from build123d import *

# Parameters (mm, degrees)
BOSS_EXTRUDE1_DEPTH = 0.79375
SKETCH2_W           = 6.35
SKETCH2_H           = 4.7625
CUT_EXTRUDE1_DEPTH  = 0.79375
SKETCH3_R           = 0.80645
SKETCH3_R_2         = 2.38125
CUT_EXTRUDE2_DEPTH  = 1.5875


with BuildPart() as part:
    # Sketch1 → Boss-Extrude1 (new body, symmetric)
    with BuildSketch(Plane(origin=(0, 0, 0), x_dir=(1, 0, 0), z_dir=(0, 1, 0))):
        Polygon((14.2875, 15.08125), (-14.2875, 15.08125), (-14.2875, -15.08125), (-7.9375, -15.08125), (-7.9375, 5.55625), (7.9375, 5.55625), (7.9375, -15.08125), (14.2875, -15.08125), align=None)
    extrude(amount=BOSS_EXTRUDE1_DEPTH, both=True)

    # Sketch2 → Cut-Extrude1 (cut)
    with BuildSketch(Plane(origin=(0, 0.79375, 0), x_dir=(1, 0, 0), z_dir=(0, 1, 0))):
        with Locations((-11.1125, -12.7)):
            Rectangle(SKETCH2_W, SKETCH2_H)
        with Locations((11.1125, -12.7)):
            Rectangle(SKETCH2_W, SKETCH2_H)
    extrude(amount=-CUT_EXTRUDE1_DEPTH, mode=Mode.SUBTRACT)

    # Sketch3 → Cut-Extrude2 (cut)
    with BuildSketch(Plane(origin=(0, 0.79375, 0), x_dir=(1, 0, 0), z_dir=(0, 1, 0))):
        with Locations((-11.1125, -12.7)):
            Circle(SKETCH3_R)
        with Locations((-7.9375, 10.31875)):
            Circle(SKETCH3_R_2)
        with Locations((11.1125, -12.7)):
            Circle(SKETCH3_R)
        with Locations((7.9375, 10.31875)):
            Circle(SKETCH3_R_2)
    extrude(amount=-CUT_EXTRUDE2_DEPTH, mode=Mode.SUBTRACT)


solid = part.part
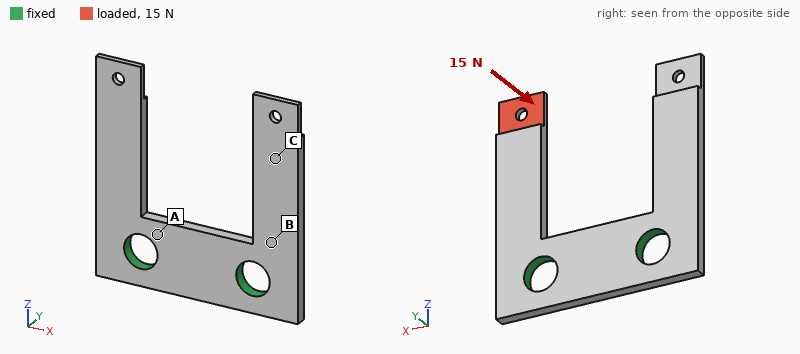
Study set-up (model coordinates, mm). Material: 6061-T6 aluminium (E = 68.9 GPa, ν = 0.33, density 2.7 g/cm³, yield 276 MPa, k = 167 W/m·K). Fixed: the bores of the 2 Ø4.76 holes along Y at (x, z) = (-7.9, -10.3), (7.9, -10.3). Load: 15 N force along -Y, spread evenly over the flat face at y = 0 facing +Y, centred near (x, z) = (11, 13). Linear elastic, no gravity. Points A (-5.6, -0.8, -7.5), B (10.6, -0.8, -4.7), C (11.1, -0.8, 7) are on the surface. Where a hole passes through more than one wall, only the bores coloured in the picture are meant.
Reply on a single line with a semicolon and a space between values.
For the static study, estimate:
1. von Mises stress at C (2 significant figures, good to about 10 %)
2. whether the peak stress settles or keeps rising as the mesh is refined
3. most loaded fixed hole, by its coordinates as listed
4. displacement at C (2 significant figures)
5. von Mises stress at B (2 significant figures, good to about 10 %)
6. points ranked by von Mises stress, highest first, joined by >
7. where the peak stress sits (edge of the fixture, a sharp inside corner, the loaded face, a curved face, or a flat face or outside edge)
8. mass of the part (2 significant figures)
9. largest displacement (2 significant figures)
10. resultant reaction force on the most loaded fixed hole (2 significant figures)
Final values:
33 MPa; keeps rising; (7.9, -10.3); 0.19 mm; 94 MPa; B > C > A; a sharp inside corner; 2.0 g; 0.39 mm; 16 N
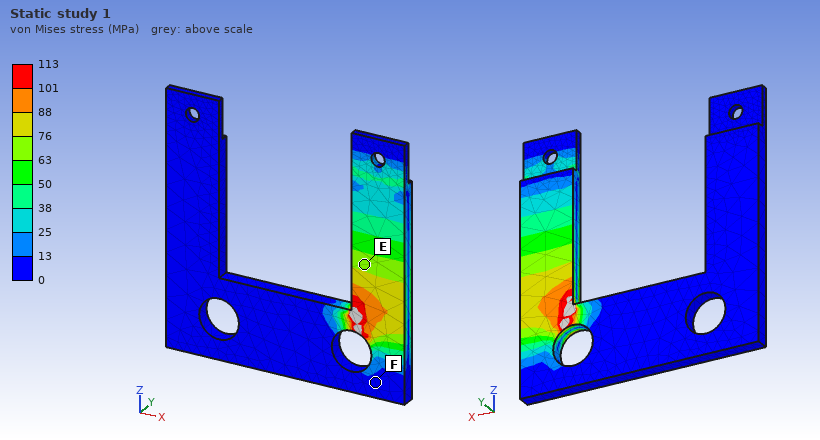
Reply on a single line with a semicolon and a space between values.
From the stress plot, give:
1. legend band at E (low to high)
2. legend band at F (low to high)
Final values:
63 to 76 MPa; 0 to 13 MPa
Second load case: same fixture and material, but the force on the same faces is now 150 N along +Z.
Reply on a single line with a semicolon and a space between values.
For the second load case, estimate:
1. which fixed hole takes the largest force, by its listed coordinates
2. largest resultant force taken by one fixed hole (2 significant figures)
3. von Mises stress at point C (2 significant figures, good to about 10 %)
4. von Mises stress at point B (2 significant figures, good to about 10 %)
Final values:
(7.9, -10.3); 150 N; 14 MPa; 15 MPa
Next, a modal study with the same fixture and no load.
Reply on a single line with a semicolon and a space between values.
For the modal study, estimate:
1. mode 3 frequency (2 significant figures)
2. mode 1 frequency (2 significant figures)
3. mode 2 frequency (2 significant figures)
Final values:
10 kHz; 2800 Hz; 2800 Hz
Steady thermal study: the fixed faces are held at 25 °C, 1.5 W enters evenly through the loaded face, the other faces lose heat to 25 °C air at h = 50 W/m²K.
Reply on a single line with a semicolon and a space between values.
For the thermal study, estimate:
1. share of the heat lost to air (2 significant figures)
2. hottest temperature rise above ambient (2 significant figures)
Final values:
11 %; 21 K
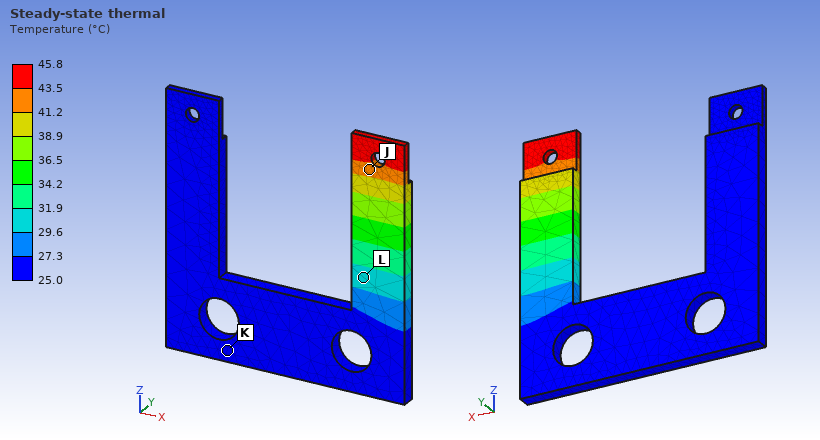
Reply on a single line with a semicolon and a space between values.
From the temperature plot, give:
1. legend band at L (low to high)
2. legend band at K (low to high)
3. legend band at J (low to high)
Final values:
29.6 to 31.9 °C; 25.0 to 27.3 °C; 41.2 to 43.5 °C
